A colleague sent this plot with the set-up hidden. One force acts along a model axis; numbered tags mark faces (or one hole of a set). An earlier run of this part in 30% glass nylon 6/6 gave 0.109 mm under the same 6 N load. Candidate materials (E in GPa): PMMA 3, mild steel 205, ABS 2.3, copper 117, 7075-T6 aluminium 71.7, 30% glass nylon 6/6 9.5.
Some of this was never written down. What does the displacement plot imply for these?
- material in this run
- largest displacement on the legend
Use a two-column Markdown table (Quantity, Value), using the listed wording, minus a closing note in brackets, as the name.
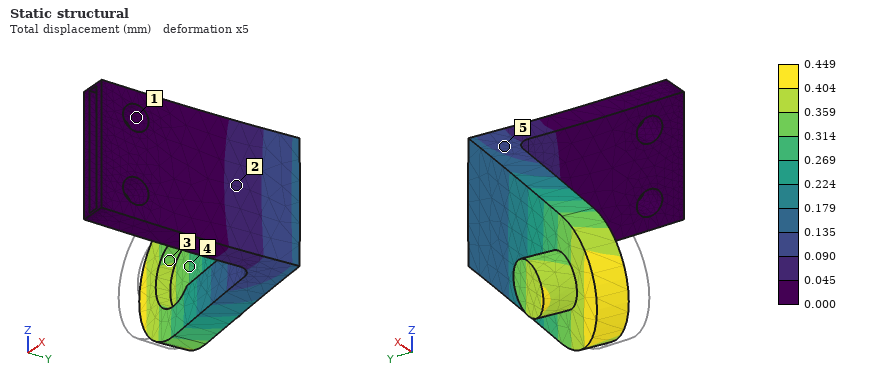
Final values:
| Quantity | Value |
|---|---|
| material in this run | ABS |
| largest displacement on the legend | 0.449 mm |
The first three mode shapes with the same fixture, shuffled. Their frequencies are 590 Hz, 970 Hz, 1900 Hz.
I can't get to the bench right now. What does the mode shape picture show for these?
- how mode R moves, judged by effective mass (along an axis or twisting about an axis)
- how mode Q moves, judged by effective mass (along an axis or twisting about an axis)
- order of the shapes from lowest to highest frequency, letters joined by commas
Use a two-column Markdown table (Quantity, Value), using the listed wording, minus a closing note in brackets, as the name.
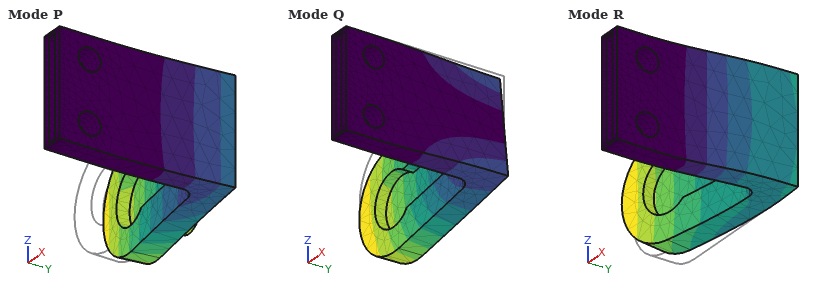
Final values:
| Quantity | Value |
|---|---|
| how mode R moves, judged by effective mass | along X |
| how mode Q moves, judged by effective mass | along Z |
| order of the shapes from lowest to highest frequency, letters joined by commas | P, Q, R |
